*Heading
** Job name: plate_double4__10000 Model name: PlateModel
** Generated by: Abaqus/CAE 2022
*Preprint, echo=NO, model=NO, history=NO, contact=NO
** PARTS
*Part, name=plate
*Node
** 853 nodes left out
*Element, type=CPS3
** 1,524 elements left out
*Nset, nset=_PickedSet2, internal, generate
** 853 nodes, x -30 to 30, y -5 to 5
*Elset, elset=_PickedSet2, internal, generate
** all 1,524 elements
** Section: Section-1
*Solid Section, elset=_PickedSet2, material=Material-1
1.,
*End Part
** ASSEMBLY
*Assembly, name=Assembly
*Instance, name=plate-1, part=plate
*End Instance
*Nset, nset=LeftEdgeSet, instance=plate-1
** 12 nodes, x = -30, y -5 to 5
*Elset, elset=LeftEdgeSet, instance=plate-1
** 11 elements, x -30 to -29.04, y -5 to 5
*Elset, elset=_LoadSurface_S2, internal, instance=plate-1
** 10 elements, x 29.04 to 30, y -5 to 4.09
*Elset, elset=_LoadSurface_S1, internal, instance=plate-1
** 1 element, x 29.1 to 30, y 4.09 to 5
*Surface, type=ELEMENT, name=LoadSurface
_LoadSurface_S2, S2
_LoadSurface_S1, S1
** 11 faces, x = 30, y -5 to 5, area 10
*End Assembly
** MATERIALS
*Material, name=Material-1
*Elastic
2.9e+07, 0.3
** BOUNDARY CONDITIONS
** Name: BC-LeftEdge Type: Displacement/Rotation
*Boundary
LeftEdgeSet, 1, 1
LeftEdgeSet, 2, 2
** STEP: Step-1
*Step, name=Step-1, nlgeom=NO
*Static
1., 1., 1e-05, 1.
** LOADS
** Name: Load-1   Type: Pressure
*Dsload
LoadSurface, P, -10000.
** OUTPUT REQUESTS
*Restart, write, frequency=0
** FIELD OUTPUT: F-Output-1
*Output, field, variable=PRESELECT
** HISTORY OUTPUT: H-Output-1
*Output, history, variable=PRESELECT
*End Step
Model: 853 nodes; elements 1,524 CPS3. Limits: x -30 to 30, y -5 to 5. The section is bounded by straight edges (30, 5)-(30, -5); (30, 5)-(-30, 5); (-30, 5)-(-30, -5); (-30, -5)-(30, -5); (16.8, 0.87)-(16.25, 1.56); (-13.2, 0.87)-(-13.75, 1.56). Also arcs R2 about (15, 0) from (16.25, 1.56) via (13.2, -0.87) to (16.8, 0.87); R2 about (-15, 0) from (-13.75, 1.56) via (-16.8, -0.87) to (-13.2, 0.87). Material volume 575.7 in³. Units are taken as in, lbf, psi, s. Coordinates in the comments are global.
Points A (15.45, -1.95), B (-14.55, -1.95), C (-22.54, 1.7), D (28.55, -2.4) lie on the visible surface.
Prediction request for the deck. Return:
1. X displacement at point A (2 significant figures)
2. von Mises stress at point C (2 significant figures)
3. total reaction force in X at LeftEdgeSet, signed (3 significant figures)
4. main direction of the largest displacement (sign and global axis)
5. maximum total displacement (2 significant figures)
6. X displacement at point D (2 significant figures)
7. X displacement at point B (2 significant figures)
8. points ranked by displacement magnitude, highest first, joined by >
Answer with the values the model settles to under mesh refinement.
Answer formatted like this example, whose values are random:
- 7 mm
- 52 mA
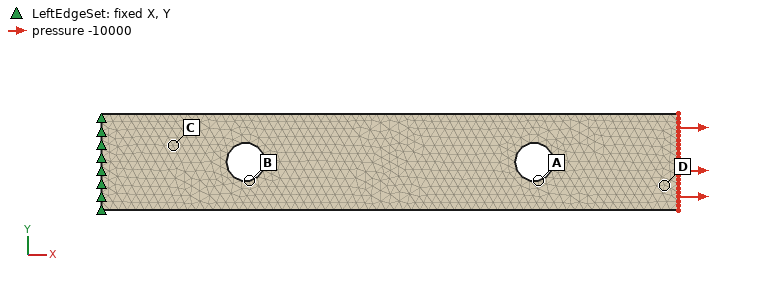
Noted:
- 0.018 in
- 9200 psi
- -1.00e+05 lbf
- +X
- 0.024 in
- 0.023 in
- 0.0064 in
- D > A > B > C
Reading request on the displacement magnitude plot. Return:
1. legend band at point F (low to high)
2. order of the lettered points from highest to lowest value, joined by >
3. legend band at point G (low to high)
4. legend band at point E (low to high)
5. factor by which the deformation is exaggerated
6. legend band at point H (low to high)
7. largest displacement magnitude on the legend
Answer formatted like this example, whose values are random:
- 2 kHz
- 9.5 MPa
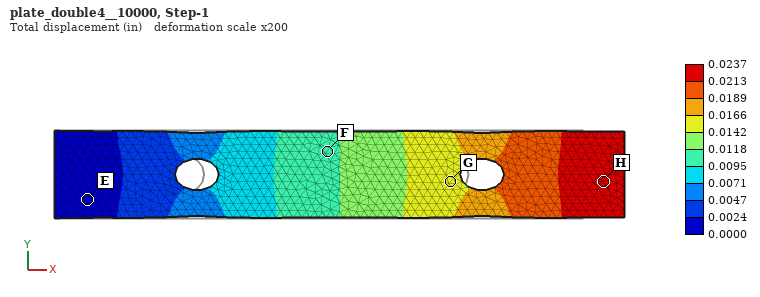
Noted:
- 0.0095 to 0.0118 in
- H > G > F > E
- 0.0142 to 0.0166 in
- 0.0000 to 0.0024 in
- 200
- 0.0213 to 0.0237 in
- 0.0237 in
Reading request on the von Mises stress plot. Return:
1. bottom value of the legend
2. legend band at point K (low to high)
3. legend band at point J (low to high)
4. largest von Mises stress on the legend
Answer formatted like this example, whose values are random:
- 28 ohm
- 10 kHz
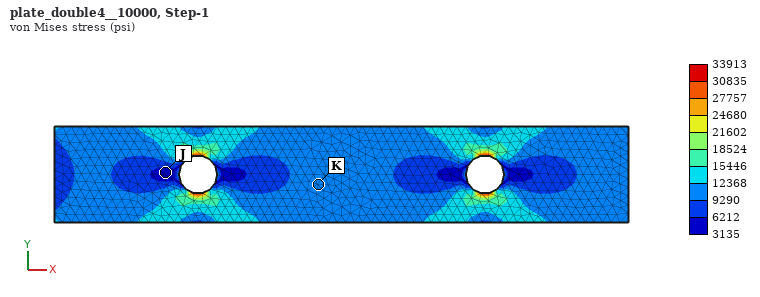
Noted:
- 3135 psi
- 9290 to 12368 psi
- 3135 to 6212 psi
- 33913 psi
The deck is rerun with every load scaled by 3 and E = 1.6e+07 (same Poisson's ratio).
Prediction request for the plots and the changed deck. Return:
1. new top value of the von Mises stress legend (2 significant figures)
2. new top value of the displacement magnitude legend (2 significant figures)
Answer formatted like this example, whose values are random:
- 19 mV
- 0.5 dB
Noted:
- 1.0e+05 psi
- 0.13 in
